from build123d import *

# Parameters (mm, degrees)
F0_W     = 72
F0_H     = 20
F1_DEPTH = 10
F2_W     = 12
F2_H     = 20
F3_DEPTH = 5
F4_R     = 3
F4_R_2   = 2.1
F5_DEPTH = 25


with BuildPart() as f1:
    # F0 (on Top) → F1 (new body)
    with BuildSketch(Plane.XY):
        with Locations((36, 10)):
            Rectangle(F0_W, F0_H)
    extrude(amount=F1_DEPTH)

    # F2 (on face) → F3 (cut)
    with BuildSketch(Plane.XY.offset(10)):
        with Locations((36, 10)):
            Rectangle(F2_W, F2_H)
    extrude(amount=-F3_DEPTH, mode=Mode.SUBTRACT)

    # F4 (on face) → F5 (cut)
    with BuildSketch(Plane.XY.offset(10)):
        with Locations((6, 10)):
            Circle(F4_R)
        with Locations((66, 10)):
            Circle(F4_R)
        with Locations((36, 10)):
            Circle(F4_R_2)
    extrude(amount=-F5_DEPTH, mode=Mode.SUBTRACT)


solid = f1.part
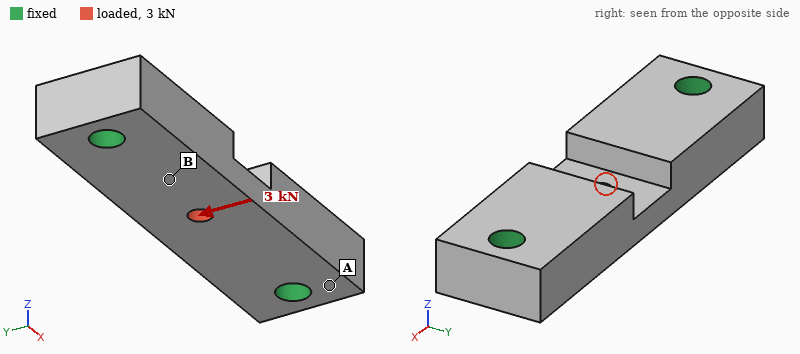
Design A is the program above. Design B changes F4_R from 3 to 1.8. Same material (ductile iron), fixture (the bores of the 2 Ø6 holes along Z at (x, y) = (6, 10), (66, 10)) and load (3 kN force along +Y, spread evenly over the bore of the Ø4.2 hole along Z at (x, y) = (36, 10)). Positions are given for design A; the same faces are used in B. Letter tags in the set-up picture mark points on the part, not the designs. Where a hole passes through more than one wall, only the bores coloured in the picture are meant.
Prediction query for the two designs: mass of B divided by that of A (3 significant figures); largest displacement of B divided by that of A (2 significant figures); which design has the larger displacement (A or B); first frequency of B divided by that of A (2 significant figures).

1.03
1.4
B
0.87
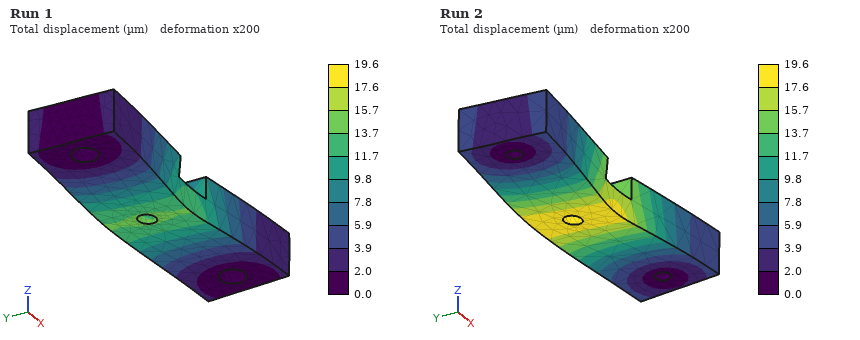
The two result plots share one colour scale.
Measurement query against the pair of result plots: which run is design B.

Run 2
